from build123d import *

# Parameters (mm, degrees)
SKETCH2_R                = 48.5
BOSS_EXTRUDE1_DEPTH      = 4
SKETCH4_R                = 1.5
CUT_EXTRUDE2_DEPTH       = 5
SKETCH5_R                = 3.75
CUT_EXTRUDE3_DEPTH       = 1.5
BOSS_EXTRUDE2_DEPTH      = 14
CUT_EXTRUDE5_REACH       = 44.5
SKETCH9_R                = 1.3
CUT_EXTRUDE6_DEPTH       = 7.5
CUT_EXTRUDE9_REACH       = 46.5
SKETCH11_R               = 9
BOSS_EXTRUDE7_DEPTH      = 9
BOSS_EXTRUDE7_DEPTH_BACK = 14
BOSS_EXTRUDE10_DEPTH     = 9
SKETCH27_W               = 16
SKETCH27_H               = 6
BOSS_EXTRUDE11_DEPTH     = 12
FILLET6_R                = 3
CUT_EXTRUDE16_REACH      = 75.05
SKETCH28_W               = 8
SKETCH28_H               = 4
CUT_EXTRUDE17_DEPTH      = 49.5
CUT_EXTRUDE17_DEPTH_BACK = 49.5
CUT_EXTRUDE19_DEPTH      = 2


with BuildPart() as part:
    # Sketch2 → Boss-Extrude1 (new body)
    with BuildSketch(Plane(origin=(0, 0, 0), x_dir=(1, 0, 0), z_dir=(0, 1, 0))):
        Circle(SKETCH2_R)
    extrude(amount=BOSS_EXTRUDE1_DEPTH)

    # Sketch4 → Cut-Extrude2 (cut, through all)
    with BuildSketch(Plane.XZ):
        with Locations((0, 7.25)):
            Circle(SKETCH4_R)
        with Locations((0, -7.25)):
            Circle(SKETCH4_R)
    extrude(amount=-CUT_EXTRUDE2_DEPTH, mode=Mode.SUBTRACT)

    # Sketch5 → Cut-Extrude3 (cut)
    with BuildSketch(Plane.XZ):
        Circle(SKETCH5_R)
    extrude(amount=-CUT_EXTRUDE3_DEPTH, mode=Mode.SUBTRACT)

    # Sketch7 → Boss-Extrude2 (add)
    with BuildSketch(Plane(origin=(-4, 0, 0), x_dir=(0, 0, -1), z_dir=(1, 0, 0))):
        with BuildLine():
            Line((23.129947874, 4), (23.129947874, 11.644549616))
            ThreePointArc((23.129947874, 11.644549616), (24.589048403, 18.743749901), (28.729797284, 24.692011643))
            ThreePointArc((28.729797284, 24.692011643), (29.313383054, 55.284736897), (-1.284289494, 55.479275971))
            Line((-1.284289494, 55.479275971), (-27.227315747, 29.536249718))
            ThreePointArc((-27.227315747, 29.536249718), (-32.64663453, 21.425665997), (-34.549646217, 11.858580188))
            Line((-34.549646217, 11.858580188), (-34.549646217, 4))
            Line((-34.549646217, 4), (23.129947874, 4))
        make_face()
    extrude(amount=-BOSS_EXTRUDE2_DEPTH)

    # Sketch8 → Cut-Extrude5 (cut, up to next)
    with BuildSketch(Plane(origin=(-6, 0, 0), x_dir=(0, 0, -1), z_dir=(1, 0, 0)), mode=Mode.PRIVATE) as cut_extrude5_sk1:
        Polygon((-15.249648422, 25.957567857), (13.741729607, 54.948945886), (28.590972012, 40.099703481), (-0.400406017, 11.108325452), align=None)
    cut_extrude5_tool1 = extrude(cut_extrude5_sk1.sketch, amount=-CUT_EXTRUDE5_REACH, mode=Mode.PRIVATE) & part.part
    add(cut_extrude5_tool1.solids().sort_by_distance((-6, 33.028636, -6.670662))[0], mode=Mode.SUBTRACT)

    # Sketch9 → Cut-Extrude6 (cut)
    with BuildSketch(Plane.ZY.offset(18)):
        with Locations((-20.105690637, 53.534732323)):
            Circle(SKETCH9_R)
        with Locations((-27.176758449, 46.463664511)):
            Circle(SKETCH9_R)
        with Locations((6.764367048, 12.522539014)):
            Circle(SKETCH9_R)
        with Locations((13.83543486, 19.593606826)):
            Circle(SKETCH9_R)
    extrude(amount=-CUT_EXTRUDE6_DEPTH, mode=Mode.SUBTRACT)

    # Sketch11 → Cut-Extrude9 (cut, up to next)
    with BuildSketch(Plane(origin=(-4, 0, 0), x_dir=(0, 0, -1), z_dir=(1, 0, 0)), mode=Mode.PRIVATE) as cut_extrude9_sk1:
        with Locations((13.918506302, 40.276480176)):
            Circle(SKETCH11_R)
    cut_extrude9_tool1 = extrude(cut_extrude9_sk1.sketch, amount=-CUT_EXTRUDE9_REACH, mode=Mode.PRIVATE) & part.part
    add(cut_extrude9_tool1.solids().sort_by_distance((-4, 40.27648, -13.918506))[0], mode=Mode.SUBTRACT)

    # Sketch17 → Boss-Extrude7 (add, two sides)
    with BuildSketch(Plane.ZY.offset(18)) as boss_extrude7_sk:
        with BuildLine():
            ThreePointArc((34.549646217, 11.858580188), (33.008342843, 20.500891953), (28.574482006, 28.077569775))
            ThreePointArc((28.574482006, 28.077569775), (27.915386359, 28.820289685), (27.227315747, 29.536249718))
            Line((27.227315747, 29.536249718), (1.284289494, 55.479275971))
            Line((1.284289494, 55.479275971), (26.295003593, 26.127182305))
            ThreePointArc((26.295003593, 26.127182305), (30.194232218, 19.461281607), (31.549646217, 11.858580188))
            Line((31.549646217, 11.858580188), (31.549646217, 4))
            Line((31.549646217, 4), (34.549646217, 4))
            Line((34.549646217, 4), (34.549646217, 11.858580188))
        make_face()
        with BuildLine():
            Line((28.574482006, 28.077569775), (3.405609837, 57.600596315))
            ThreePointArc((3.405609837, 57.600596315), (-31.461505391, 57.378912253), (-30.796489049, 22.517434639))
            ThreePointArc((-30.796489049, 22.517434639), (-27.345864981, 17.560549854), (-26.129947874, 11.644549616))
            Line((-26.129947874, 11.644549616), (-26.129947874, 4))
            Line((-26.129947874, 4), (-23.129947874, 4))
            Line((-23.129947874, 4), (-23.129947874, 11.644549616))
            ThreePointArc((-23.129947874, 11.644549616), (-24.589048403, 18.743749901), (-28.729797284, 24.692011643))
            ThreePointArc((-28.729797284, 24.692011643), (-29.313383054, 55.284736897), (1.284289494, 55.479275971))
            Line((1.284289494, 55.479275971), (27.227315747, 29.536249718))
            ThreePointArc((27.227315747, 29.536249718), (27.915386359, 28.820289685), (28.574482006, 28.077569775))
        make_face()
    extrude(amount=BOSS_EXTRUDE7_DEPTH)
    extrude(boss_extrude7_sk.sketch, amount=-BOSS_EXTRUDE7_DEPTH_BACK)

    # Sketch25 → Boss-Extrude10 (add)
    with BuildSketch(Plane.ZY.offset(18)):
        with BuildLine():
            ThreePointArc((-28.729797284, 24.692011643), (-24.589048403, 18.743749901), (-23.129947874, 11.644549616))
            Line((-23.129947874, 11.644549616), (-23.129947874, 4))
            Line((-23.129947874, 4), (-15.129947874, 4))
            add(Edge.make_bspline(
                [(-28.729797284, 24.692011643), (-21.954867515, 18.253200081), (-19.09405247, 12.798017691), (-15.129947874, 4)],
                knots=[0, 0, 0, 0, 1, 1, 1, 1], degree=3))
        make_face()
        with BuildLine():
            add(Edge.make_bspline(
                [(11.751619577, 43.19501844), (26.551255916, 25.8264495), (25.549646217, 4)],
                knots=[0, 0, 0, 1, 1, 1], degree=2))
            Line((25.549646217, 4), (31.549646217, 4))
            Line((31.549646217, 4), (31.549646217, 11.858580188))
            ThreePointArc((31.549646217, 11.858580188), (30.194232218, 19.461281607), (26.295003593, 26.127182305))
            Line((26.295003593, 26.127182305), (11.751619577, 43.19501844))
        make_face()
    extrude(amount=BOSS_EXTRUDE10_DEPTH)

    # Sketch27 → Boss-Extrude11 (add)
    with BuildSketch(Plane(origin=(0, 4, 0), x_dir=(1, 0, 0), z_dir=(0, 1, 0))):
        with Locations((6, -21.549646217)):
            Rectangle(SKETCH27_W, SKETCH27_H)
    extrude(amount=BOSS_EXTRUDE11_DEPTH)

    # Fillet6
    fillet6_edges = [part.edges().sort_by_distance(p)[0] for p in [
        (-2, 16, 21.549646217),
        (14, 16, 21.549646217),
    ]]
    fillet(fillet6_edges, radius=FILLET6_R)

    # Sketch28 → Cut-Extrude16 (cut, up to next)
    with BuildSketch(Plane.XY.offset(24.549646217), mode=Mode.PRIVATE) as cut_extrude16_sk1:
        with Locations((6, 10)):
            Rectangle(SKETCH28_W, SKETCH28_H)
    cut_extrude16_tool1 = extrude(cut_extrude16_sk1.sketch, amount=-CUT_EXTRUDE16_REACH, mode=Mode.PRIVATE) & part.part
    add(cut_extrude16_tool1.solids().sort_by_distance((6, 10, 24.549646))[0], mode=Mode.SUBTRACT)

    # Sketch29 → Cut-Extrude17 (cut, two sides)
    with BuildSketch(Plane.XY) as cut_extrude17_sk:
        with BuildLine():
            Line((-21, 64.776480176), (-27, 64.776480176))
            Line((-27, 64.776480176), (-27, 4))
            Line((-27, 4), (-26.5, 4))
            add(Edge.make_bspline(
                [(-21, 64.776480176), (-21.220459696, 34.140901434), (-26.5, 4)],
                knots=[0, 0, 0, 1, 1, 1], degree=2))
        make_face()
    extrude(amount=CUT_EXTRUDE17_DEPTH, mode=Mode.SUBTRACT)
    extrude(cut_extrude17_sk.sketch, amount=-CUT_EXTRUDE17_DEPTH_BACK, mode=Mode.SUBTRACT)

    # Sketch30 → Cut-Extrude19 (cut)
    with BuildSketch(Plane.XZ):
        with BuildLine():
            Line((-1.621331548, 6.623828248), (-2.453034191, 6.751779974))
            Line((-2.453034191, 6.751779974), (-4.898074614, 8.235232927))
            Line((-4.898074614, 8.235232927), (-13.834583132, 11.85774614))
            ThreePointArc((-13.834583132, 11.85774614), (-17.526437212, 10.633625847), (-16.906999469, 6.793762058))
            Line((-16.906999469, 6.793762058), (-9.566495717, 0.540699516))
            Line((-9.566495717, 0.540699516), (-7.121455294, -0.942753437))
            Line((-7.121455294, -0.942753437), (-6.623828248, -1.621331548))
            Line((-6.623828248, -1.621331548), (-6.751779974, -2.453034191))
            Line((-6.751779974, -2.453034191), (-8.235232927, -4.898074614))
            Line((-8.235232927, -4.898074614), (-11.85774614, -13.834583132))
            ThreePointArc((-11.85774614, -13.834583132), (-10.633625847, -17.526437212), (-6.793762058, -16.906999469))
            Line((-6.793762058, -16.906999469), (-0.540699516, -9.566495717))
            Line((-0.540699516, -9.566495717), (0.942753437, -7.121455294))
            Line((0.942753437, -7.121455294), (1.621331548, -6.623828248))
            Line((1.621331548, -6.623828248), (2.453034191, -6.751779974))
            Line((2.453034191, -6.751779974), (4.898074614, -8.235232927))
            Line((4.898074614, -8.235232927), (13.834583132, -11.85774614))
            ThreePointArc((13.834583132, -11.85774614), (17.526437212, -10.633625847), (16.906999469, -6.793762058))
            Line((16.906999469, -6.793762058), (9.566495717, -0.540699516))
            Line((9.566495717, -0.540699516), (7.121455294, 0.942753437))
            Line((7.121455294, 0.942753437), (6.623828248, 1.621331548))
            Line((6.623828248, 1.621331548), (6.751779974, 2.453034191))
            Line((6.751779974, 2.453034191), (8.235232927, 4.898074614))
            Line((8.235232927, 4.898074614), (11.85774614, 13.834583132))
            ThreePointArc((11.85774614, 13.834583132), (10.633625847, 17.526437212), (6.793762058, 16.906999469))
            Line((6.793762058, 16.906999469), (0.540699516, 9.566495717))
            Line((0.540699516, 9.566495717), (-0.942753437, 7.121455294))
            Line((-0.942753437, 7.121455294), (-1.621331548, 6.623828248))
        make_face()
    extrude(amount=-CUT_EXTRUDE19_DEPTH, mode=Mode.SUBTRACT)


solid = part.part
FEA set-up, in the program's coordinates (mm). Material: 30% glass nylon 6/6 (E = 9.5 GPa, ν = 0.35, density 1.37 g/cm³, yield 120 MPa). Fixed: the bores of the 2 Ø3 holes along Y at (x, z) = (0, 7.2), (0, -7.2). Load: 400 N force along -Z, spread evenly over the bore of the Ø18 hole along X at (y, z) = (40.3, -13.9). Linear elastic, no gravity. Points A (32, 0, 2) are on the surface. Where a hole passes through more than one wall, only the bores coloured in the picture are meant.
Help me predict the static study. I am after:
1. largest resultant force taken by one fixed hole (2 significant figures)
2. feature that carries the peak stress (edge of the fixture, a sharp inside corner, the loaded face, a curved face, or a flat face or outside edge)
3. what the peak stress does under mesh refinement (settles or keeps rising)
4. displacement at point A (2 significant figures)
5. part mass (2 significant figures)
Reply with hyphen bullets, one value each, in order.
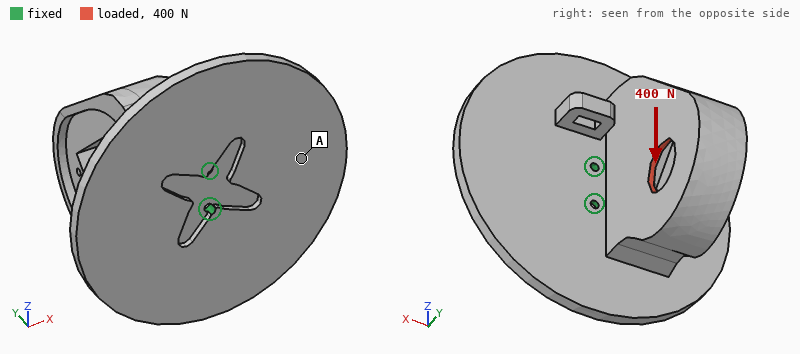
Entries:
- 780 N
- edge of the fixture
- keeps rising
- 0.14 mm
- 92 g
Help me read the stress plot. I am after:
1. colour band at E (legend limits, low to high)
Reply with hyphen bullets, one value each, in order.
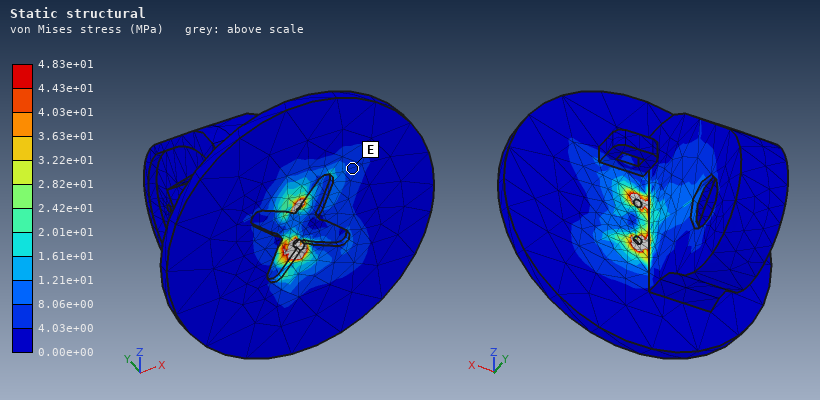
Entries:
- 4.03e+00 to 8.06e+00 MPa
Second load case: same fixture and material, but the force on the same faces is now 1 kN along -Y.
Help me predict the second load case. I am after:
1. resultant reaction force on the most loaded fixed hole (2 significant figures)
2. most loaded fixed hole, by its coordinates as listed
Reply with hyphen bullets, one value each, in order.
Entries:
- 1.2 kN
- (0, -7.2)
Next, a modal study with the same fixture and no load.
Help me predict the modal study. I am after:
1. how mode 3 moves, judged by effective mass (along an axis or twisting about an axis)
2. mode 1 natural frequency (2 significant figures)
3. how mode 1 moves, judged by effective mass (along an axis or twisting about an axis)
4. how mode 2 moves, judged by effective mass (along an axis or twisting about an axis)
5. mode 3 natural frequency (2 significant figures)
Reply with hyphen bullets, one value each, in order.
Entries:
- along Y
- 240 Hz
- along X
- along Z
- 780 Hz
